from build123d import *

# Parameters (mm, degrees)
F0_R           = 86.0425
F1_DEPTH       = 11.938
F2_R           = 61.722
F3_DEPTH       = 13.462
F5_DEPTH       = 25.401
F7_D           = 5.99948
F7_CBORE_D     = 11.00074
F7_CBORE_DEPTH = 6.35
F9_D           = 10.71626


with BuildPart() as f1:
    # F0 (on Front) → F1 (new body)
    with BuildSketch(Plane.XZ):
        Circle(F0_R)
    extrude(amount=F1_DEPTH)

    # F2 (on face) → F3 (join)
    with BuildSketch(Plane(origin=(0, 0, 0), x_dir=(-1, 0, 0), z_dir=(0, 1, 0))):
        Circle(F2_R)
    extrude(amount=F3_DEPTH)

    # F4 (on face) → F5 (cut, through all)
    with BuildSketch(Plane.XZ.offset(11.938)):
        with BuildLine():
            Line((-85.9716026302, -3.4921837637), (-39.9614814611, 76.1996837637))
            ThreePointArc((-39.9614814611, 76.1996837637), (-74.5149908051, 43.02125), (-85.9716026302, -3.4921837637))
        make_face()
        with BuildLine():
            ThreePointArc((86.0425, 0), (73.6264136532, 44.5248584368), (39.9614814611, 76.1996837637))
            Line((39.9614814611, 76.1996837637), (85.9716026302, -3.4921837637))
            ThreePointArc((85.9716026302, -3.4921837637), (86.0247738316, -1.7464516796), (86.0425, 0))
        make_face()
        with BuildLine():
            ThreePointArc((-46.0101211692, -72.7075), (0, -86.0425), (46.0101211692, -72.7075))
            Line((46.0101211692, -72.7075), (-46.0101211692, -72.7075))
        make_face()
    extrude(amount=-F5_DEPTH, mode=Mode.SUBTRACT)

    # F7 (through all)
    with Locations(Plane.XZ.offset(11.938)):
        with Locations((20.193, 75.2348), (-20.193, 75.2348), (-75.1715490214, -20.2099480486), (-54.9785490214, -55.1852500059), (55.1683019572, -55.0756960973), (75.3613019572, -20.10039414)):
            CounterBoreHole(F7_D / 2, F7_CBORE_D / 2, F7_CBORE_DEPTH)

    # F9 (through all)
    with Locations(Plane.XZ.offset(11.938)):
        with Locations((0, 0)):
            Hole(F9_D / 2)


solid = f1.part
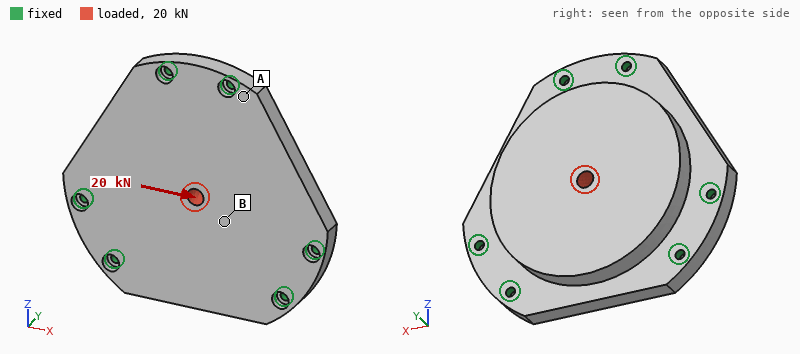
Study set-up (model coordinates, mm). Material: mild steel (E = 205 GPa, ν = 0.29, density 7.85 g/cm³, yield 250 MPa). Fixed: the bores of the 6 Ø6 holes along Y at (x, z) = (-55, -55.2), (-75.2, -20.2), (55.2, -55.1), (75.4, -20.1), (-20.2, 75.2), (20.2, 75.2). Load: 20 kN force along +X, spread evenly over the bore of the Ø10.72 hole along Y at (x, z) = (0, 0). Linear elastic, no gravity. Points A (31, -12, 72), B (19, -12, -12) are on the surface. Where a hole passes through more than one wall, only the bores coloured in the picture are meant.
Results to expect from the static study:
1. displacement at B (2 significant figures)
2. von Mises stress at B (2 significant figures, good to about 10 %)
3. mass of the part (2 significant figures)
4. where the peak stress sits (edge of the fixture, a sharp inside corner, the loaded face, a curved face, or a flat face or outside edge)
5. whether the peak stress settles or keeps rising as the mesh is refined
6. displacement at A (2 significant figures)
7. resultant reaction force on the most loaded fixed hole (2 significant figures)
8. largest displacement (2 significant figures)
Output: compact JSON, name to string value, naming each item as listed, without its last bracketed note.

{"displacement at B": "3.8 µm", "von Mises stress at B": "11 MPa", "mass of the part": "3.2 kg", "where the peak stress sits": "edge of the fixture", "whether the peak stress settles or keeps rising as the mesh is refined": "keeps rising", "displacement at A": "1.4 µm", "resultant reaction force on the most loaded fixed hole": "4.2 kN", "largest displacement": "6.1 µm"}
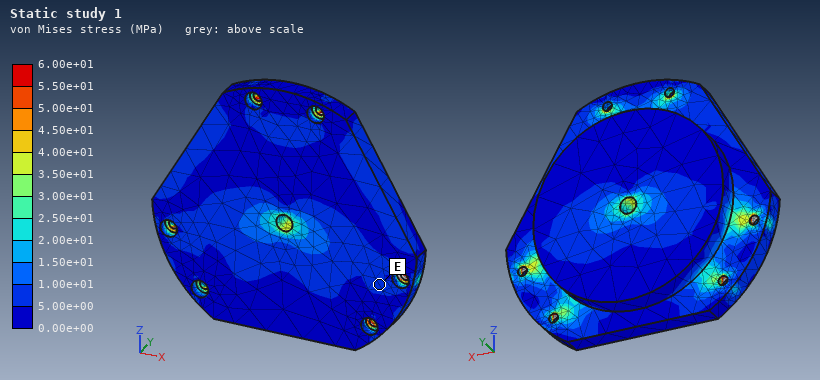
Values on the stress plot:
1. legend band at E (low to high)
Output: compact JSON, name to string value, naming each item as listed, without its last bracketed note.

{"legend band at E": "5.00e+00 to 1.00e+01 MPa"}
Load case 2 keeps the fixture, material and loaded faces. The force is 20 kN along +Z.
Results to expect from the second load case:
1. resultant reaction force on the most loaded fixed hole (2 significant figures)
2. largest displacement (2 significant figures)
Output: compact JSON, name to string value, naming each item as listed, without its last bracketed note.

{"resultant reaction force on the most loaded fixed hole": "4.2 kN", "largest displacement": "6.2 µm"}
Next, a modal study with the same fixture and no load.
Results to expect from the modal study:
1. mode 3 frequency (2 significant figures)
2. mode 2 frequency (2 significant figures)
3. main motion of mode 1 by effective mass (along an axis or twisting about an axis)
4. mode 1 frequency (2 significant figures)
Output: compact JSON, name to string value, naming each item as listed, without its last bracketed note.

{"mode 3 frequency": "4800 Hz", "mode 2 frequency": "4800 Hz", "main motion of mode 1 by effective mass": "along Y", "mode 1 frequency": "3200 Hz"}
